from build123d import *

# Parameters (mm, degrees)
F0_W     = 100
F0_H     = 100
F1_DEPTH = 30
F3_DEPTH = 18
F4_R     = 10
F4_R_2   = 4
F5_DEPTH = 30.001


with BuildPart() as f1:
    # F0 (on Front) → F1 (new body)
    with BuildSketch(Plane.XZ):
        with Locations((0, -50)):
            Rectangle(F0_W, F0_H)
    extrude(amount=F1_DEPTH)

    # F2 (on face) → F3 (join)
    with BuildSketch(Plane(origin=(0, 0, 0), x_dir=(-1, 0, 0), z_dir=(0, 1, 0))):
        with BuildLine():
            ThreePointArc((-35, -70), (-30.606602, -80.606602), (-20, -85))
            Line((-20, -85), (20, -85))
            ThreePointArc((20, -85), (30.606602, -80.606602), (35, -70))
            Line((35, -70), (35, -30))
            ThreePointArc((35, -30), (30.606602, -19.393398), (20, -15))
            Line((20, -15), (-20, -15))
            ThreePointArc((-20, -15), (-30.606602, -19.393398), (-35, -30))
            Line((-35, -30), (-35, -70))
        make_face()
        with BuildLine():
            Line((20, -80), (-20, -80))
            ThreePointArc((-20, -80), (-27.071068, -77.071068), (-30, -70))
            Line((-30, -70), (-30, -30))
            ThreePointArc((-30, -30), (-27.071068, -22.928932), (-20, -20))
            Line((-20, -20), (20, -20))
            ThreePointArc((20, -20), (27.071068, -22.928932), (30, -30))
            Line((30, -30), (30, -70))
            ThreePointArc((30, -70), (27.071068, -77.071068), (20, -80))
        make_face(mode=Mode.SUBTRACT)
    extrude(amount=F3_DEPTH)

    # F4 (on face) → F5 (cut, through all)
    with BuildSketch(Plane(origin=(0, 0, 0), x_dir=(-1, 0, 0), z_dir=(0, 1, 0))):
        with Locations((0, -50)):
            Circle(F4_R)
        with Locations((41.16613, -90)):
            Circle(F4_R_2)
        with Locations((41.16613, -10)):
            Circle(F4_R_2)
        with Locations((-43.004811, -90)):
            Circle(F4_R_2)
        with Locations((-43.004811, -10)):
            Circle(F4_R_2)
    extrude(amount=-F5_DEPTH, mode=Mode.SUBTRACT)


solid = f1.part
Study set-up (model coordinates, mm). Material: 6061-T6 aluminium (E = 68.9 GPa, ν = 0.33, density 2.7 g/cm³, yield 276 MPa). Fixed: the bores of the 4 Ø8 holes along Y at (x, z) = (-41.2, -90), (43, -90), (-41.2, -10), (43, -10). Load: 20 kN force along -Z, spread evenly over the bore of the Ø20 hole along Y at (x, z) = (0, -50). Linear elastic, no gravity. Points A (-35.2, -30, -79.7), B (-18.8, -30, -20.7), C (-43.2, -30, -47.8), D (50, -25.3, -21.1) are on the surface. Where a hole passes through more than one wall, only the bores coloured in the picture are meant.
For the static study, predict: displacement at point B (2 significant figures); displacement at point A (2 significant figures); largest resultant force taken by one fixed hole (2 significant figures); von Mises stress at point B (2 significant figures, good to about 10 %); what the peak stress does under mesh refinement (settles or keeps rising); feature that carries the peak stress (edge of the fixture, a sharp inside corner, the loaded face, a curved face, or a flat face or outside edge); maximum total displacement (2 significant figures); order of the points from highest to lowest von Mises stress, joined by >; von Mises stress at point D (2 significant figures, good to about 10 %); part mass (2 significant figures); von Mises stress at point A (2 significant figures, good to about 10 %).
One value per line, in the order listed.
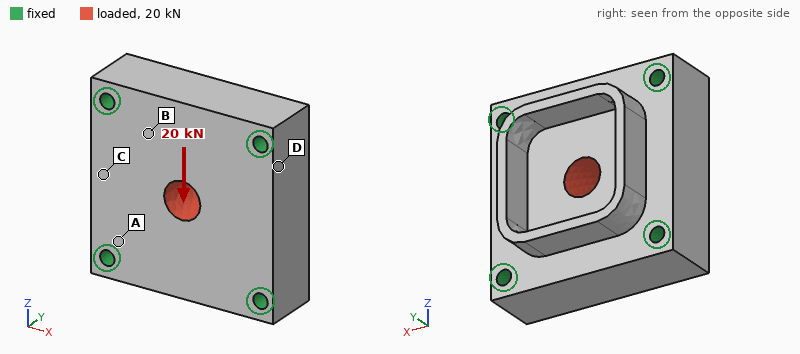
4.2 µm
1.4 µm
5.8 kN
7.1 MPa
keeps rising
edge of the fixture
7.8 µm
A > B > D > C
3.8 MPa
830 g
9.0 MPa
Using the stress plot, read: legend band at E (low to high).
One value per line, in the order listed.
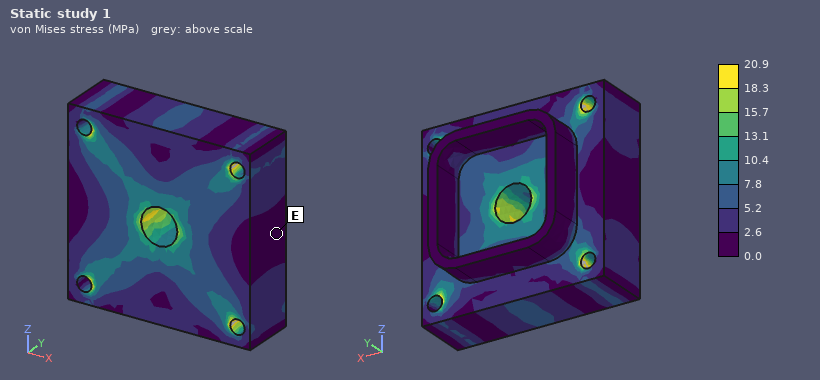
0.0 to 2.6 MPa
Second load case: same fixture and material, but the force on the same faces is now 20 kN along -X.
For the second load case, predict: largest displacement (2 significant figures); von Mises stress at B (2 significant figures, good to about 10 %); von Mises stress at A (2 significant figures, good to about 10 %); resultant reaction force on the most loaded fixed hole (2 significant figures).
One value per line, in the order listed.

7.5 µm
6.5 MPa
8.6 MPa
5.7 kN
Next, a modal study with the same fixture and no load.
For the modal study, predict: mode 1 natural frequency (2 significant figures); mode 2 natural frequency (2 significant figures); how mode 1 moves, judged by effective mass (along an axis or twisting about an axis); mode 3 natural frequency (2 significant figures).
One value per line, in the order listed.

9800 Hz
12 kHz
along Y
13 kHz
